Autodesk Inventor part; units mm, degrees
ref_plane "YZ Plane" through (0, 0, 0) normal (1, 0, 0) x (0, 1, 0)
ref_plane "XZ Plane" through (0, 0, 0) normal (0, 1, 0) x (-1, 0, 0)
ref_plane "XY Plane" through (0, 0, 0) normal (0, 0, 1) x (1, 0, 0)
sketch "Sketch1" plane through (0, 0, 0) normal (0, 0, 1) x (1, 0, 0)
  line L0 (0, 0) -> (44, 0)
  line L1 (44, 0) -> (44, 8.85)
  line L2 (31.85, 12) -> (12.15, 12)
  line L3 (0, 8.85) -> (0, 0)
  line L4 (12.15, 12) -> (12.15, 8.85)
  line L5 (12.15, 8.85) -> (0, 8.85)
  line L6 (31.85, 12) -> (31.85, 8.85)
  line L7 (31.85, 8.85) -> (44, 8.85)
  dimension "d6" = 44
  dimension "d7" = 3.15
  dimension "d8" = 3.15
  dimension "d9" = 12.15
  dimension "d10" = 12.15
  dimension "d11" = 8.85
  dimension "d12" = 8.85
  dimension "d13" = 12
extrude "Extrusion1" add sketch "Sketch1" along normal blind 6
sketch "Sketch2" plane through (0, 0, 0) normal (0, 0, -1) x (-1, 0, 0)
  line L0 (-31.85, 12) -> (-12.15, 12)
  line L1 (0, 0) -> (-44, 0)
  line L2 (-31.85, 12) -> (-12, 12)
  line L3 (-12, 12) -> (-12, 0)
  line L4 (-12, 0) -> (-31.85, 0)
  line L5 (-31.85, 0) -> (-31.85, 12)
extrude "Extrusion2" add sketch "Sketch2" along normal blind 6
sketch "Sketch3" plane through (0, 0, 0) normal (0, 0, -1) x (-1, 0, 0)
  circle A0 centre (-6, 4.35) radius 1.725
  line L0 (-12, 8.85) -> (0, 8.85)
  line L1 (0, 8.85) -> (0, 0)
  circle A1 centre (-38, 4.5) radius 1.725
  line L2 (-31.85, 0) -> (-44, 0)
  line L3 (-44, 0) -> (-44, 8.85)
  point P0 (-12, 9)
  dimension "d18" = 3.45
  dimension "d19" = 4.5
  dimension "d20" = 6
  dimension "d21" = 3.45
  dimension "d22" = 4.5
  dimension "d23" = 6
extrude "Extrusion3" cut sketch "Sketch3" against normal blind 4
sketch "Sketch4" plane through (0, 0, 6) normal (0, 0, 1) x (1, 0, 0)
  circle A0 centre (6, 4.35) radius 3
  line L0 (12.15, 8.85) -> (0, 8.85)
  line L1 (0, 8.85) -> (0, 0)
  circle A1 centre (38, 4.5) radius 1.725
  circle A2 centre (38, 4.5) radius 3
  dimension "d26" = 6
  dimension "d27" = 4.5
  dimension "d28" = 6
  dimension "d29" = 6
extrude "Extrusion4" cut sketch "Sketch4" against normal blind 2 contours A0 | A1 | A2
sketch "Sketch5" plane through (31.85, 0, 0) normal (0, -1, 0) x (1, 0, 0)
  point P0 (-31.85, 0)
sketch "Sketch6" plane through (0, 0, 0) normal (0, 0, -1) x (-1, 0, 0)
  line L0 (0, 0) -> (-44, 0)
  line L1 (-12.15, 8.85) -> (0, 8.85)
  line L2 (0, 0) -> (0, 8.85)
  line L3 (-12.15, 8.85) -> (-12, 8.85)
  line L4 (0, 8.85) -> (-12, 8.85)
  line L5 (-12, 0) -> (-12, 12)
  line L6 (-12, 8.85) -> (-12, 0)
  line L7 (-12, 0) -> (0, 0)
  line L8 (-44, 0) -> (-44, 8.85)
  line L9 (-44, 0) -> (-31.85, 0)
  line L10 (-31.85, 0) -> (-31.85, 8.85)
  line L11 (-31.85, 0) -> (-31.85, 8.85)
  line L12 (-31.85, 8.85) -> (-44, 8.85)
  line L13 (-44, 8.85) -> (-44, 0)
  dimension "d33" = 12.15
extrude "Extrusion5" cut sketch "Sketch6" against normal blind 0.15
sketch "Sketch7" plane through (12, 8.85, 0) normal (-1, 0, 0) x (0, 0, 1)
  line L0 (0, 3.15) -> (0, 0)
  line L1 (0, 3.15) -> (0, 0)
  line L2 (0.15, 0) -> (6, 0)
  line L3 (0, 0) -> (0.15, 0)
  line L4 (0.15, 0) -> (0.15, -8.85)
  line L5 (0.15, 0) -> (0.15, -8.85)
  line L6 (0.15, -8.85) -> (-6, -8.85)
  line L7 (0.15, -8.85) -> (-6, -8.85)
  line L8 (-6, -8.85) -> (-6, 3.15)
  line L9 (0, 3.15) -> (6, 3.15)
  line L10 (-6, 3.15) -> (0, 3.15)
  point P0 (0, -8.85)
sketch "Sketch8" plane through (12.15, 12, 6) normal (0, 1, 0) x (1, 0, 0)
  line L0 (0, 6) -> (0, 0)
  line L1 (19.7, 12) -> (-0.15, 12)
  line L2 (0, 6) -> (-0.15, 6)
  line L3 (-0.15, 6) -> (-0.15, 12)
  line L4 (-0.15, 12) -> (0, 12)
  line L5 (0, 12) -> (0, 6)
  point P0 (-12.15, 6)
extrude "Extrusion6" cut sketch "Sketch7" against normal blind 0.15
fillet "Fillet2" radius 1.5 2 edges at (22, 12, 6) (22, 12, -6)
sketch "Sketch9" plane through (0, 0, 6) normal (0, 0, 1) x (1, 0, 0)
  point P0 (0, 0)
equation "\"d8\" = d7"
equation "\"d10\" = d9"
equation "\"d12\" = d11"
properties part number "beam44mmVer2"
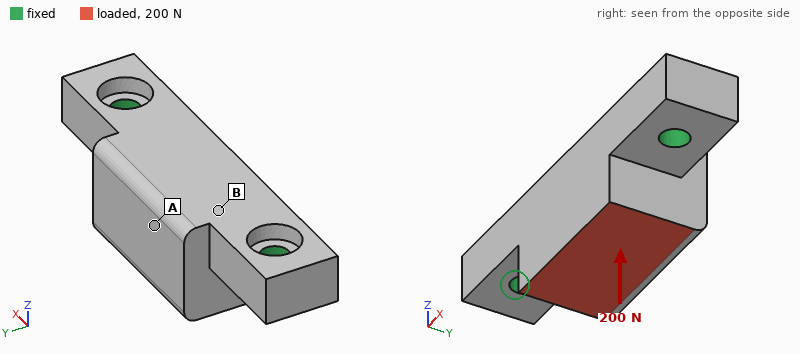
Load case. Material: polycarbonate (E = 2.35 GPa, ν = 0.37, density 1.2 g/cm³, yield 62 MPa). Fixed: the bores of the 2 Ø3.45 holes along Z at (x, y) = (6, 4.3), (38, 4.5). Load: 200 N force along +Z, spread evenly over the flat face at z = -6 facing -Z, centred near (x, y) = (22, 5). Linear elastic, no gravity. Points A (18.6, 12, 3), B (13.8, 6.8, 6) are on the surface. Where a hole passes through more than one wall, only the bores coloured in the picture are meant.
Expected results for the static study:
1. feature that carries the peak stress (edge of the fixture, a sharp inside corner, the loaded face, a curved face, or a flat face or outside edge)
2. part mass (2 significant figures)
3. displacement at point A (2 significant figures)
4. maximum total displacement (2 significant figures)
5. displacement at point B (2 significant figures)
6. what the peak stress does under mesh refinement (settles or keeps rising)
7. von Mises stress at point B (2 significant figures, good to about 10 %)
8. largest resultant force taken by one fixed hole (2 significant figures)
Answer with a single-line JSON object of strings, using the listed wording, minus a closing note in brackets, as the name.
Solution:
{"feature that carries the peak stress": "edge of the fixture", "part mass": "4.7 g", "displacement at point A": "68 µm", "maximum total displacement": "71 µm", "displacement at point B": "46 µm", "what the peak stress does under mesh refinement": "keeps rising", "von Mises stress at point B": "4.8 MPa", "largest resultant force taken by one fixed hole": "100 N"}
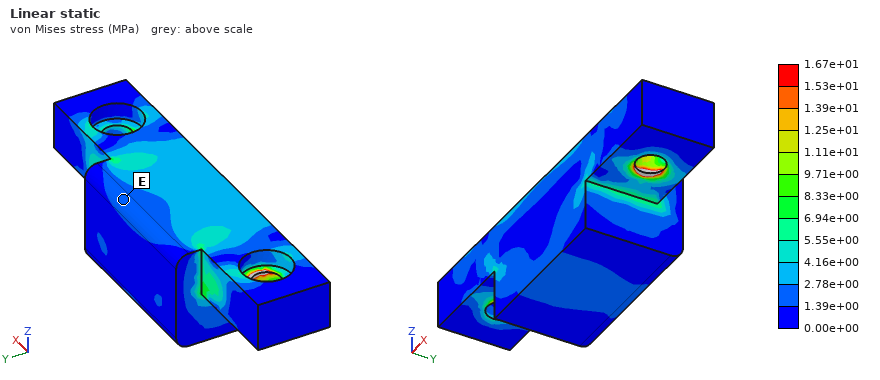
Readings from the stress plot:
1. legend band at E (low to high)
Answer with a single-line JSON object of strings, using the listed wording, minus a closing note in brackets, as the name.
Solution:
{"legend band at E": "1.39e+00 to 2.78e+00 MPa"}
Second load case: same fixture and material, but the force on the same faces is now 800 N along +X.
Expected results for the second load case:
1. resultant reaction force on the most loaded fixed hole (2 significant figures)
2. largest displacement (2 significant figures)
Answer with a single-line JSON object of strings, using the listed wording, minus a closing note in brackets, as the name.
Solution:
{"resultant reaction force on the most loaded fixed hole": "470 N", "largest displacement": "0.17 mm"}
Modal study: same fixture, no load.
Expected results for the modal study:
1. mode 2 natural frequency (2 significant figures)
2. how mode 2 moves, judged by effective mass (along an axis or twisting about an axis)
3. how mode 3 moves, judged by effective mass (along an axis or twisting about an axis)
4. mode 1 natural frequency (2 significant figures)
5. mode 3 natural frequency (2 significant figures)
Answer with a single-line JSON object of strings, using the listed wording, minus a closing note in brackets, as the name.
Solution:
{"mode 2 natural frequency": "5600 Hz", "how mode 2 moves, judged by effective mass": "along Z", "how mode 3 moves, judged by effective mass": "along Y", "mode 1 natural frequency": "3500 Hz", "mode 3 natural frequency": "7200 Hz"}
